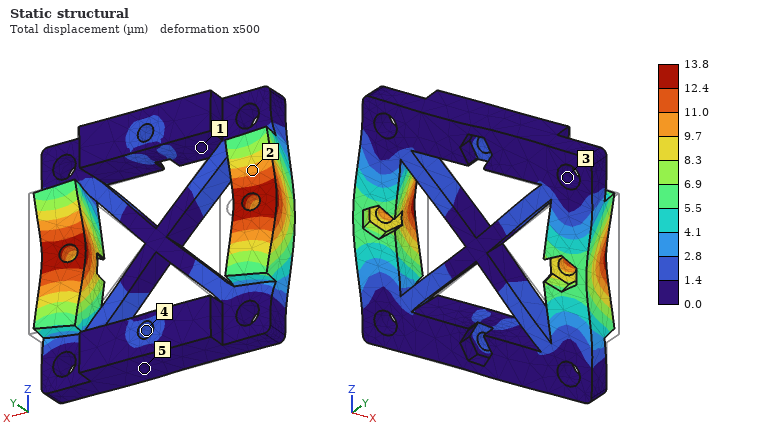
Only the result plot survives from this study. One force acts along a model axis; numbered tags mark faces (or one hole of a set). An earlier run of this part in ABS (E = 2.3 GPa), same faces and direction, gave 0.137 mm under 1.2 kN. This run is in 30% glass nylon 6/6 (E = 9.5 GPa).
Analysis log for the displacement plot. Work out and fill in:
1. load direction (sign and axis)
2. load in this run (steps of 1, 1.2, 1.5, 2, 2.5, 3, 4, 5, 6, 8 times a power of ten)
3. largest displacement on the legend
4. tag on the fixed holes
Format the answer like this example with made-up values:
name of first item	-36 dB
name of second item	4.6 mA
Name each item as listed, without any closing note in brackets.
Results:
load direction	-X
load in this run	500 N
largest displacement on the legend	13.8 µm
tag on the fixed holes	3
